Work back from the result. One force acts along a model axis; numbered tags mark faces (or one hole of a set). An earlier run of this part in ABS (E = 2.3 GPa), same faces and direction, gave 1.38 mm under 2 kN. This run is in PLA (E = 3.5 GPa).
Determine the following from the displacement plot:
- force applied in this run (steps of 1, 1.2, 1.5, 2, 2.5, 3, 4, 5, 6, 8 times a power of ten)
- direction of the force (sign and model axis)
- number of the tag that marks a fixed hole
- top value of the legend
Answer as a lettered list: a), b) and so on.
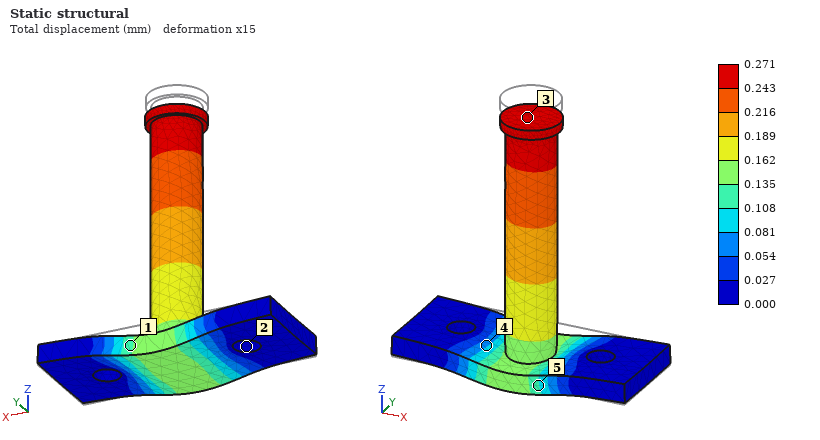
a) 600 N
b) -Z
c) 2
d) 0.271 mm
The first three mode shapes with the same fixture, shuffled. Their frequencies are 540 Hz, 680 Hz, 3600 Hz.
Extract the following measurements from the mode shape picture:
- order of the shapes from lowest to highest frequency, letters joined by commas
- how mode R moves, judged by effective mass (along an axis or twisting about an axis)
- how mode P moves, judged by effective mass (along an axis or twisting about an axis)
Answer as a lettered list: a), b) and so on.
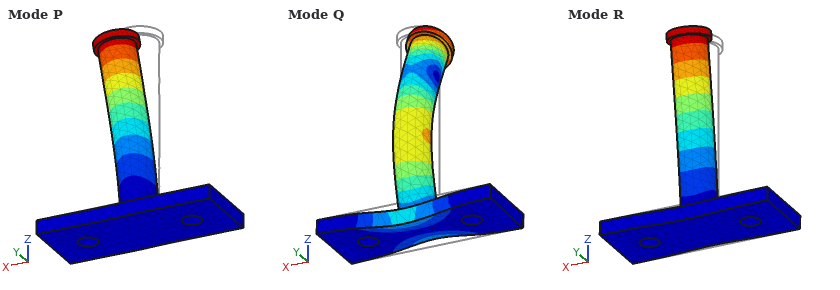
a) R, P, Q
b) along Y
c) along X
